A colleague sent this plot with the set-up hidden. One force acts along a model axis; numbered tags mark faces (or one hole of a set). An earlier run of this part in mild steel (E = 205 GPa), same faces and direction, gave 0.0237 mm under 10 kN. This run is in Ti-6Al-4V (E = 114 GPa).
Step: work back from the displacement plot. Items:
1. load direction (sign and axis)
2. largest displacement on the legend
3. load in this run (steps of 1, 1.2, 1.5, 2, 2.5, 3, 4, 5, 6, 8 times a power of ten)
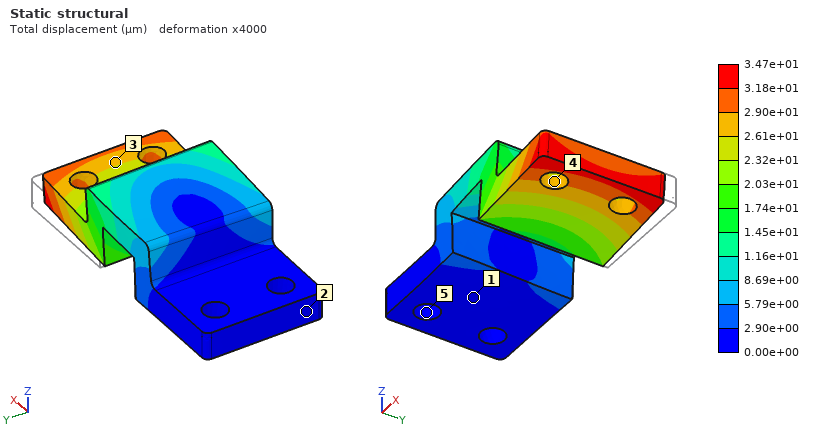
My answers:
-Y
3.47e+01 µm
8 kN
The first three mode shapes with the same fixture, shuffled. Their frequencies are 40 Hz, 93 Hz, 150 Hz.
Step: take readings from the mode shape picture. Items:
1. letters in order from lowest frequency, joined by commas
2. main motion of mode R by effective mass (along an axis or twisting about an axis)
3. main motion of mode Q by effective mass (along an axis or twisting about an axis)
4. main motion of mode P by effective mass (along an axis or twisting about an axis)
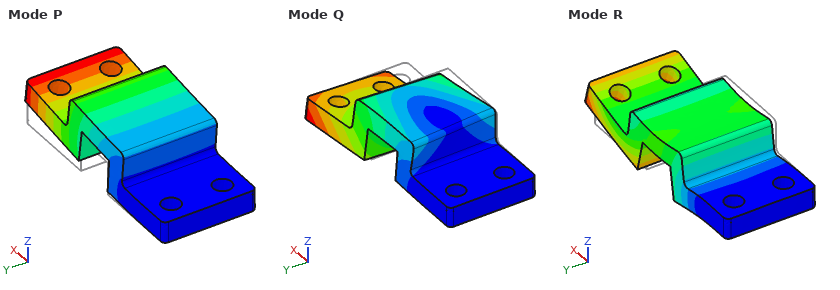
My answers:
P, Q, R
along X
along Y
along Z
